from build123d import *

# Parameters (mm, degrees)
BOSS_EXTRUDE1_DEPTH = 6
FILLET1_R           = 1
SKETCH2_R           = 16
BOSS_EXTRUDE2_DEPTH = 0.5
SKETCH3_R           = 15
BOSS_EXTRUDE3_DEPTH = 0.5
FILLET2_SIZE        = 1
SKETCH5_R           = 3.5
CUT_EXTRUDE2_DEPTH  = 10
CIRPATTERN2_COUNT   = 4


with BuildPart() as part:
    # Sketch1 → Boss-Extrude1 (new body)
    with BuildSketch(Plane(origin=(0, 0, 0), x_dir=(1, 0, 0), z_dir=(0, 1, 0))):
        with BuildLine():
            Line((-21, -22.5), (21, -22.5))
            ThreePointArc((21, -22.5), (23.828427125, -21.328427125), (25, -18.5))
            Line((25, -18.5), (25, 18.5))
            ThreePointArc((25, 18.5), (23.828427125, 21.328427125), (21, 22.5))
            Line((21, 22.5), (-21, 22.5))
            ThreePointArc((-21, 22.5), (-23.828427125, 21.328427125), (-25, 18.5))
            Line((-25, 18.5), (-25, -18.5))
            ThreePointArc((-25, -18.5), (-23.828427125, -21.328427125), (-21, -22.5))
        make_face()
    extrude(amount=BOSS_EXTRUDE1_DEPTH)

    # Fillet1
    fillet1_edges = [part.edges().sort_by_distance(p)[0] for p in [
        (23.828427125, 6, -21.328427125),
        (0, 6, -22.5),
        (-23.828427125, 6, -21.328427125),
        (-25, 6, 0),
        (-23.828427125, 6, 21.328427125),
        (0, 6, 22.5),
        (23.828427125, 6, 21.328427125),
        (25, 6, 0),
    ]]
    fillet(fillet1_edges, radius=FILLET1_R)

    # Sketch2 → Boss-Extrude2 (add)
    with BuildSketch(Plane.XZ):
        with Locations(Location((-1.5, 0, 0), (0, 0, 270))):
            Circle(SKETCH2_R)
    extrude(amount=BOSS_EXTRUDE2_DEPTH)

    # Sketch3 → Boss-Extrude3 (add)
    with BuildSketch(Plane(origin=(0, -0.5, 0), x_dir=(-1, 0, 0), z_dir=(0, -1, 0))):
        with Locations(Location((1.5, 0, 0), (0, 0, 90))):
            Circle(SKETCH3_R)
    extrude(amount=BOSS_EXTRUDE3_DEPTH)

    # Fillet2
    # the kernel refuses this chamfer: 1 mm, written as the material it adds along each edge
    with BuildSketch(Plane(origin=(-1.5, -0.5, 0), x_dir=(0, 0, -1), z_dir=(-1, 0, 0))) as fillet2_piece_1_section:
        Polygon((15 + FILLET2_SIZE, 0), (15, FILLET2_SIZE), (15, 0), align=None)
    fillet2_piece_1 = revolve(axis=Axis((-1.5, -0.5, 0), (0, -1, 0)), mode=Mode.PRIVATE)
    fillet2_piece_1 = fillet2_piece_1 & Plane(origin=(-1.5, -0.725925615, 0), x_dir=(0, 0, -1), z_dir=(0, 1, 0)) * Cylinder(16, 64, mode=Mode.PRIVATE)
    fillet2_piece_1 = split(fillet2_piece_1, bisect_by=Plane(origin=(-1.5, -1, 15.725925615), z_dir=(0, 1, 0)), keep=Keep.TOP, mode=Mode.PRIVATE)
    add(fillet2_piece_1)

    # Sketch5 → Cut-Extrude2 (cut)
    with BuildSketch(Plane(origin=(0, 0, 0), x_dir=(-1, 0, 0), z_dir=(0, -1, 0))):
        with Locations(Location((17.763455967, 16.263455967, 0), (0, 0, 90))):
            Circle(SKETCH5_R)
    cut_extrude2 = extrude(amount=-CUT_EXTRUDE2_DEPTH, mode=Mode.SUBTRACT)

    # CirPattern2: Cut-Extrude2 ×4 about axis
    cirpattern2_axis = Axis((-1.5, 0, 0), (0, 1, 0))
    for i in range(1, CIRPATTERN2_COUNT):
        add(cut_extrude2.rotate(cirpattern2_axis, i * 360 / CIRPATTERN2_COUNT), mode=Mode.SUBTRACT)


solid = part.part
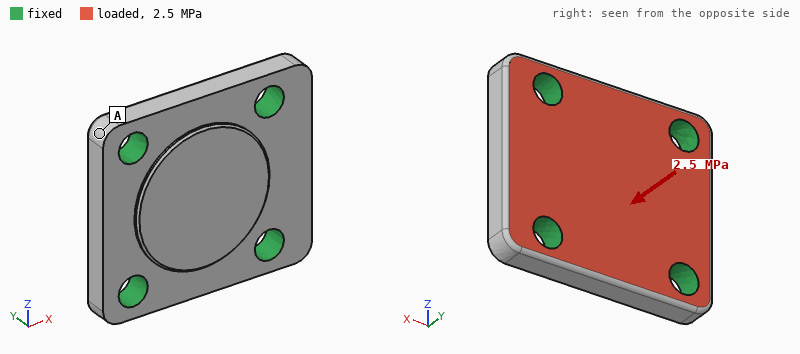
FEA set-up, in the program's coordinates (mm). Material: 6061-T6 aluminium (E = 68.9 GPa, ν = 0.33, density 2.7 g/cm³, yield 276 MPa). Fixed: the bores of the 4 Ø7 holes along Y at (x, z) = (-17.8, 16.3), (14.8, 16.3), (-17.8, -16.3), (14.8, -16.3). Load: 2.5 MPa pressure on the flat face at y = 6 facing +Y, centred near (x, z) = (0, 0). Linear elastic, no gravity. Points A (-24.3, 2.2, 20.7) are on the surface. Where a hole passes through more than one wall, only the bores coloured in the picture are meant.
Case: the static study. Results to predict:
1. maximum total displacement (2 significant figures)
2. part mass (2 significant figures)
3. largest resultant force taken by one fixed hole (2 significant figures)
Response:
9.2 µm
36 g
1.3 kN
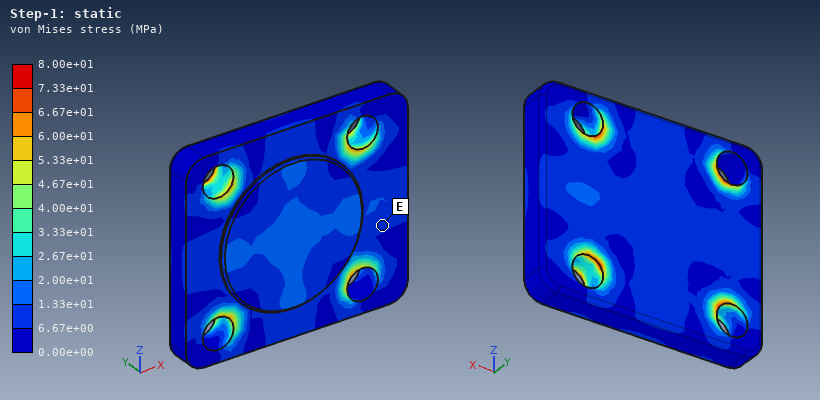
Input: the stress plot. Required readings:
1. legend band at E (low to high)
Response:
6.67e+00 to 1.33e+01 MPa
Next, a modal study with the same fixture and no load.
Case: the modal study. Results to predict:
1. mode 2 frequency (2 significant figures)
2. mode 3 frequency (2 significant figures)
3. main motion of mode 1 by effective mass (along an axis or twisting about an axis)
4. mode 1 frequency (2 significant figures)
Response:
29 kHz
34 kHz
along Y
23 kHz
